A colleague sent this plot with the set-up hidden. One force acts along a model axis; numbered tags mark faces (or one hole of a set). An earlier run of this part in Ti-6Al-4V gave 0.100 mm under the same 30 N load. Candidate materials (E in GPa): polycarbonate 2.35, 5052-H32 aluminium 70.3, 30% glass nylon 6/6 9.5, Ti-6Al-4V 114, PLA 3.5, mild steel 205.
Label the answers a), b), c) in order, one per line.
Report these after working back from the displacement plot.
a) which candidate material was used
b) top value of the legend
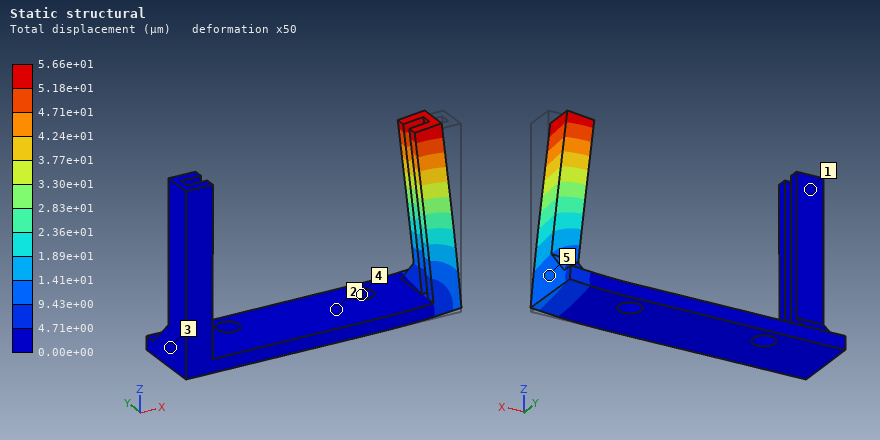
a) mild steel
b) 5.66e+01 µm
